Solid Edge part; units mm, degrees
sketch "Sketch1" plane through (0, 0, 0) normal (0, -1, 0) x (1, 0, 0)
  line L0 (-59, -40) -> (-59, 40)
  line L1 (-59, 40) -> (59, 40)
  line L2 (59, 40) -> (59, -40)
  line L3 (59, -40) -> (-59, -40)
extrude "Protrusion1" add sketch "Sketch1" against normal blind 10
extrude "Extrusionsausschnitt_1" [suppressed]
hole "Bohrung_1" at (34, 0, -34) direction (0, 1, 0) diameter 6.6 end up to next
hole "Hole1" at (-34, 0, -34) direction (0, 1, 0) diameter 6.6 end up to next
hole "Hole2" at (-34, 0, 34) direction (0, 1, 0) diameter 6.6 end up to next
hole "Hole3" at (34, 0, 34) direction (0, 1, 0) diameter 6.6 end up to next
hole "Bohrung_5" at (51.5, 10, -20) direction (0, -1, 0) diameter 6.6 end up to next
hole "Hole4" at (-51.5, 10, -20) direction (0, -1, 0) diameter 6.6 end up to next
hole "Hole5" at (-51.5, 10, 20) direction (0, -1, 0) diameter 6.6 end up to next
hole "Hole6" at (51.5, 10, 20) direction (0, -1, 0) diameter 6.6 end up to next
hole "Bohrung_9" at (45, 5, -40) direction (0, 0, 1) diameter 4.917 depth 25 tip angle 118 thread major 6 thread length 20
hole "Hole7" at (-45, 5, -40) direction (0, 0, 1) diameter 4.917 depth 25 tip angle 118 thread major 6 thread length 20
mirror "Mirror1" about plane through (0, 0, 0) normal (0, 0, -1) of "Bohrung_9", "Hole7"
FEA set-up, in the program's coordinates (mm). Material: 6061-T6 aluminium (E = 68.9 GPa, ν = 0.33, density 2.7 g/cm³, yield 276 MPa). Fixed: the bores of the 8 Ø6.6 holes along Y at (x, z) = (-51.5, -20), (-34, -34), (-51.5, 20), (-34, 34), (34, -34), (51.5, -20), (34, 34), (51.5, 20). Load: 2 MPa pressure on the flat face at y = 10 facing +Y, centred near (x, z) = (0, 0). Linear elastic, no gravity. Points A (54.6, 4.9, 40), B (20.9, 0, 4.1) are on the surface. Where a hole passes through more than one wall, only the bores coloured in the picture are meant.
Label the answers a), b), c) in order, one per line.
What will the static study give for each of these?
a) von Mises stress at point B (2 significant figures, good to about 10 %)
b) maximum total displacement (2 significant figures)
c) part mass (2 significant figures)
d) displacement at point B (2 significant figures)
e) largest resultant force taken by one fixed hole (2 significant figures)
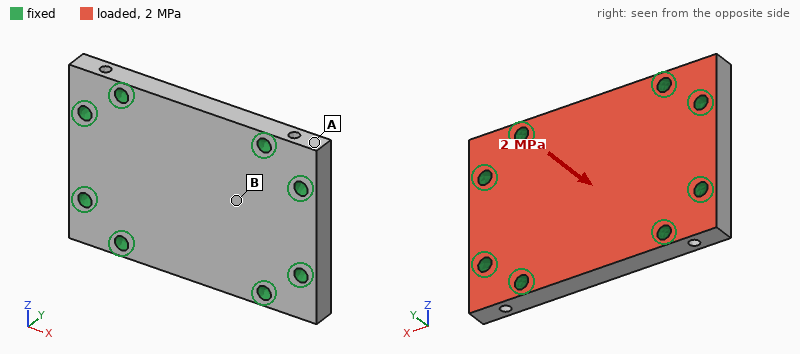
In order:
a) 20 MPa
b) 49 µm
c) 240 g
d) 36 µm
e) 3.0 kN
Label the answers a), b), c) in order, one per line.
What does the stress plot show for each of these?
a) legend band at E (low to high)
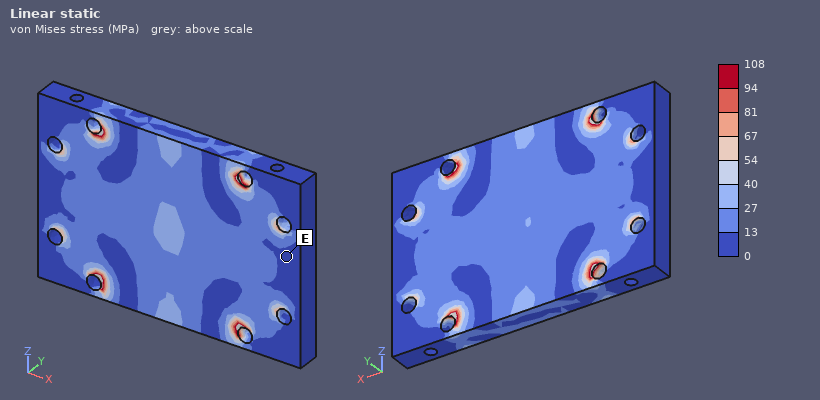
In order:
a) 0 to 13 MPa
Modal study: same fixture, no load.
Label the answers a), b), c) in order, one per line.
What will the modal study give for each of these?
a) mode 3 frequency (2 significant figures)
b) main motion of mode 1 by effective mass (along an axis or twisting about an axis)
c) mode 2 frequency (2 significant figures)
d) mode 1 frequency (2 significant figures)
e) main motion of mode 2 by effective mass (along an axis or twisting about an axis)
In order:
a) 15 kHz
b) along Y
c) 11 kHz
d) 7500 Hz
e) twisting about X
